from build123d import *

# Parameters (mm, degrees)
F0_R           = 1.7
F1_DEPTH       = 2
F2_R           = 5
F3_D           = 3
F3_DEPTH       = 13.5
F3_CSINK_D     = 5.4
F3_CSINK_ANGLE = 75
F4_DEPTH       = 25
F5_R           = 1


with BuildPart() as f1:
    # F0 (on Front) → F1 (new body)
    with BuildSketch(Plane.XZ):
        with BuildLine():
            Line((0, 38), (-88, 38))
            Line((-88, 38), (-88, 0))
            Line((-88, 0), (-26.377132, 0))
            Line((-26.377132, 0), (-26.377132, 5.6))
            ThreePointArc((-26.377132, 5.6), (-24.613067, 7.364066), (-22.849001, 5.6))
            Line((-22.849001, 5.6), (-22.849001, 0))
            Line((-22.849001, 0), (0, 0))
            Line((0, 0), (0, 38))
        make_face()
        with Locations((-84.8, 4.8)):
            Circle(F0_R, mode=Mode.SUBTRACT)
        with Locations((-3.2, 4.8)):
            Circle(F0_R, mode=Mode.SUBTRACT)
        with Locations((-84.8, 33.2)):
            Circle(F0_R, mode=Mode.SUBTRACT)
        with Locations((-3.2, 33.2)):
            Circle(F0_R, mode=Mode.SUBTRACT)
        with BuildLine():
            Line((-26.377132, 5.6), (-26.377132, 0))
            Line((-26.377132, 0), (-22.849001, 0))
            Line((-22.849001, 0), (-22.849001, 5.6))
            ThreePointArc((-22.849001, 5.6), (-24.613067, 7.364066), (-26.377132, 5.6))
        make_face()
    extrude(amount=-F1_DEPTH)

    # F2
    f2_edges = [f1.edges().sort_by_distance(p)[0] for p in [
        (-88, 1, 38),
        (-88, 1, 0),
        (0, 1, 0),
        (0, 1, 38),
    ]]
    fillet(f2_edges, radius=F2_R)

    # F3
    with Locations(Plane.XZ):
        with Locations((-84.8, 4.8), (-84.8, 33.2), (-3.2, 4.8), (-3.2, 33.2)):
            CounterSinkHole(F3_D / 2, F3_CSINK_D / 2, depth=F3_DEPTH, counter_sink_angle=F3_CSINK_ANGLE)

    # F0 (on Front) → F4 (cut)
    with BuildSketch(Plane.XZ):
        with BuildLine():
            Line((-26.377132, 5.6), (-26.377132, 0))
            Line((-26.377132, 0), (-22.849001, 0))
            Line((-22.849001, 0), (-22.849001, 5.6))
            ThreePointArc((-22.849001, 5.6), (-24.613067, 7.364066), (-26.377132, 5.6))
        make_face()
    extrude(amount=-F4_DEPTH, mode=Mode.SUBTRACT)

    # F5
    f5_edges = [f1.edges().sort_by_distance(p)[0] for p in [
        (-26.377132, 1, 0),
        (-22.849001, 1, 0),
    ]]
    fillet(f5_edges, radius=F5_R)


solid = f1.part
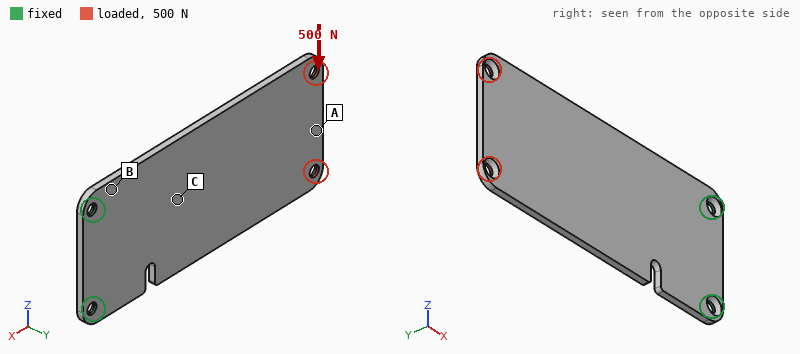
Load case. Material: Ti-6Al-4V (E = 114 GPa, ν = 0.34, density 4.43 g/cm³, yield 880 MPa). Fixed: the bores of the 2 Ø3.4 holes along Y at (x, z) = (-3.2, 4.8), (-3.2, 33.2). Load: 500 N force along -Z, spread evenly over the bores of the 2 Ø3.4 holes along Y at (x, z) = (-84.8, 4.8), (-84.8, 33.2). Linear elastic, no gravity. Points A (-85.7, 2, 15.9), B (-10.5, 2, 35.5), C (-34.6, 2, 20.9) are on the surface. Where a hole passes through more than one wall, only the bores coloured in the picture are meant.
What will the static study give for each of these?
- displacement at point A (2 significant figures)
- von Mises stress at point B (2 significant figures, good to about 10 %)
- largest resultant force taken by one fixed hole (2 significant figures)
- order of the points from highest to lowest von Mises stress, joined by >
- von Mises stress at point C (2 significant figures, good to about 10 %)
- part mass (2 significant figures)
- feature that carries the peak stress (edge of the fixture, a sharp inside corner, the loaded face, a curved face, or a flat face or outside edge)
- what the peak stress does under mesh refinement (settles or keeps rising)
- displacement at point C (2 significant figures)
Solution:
0.16 mm
92 MPa
1.4 kN
B > C > A
41 MPa
29 g
edge of the fixture
keeps rising
0.039 mm
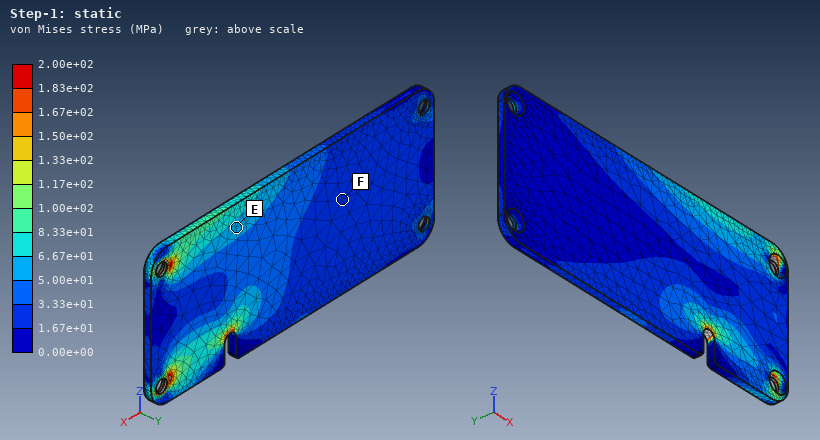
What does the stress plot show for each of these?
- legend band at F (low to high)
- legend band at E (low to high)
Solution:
1.67e+01 to 3.33e+01 MPa
5.00e+01 to 6.67e+01 MPa
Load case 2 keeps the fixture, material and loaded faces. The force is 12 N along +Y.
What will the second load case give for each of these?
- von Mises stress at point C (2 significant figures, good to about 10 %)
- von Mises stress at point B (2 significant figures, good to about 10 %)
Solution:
25 MPa
42 MPa
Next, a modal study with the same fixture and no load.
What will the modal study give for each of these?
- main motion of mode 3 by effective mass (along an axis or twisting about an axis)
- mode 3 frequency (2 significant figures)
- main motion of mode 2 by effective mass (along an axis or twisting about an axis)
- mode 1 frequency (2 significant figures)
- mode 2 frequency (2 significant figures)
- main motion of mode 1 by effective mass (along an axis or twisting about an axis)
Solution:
along Y
1300 Hz
twisting about X
200 Hz
1000 Hz
along Y
